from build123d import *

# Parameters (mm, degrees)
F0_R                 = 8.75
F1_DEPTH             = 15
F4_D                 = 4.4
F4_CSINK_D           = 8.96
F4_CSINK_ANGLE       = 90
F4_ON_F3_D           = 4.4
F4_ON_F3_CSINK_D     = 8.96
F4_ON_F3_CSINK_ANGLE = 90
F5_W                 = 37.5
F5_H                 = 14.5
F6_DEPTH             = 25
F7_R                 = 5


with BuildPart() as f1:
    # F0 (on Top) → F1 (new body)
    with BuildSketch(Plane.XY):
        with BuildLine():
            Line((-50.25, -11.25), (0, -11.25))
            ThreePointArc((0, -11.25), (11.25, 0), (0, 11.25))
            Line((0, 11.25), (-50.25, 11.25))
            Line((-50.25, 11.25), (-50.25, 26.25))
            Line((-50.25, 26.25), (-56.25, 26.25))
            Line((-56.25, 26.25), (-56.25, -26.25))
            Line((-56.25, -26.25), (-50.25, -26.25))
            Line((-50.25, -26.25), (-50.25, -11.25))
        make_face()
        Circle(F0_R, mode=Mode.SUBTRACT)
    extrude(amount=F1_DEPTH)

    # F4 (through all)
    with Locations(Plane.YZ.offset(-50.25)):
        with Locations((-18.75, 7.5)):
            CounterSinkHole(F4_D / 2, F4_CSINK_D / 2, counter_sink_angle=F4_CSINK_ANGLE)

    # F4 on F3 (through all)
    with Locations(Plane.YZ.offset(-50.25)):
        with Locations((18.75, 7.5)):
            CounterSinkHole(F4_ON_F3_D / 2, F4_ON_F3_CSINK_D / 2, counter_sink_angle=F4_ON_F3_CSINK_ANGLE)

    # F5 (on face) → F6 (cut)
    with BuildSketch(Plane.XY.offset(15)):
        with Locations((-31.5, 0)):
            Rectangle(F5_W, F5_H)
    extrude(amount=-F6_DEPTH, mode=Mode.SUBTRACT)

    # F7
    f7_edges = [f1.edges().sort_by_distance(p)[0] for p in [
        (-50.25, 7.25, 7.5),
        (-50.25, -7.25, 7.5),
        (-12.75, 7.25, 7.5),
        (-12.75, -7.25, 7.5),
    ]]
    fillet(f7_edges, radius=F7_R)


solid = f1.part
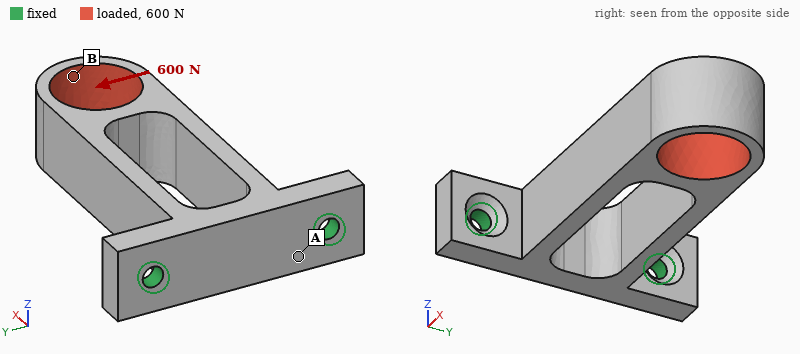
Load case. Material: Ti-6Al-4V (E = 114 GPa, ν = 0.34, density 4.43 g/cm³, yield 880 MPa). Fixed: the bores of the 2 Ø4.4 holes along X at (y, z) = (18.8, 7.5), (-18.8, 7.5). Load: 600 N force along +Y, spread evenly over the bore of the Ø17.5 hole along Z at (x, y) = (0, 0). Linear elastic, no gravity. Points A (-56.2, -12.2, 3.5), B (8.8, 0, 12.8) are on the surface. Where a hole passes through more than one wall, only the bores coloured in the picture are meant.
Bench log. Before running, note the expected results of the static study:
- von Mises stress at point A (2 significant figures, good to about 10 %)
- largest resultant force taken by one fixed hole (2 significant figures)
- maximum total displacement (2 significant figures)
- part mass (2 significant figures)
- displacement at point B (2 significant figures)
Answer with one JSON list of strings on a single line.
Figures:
["32 MPa", "1.1 kN", "0.20 mm", "57 g", "0.20 mm"]
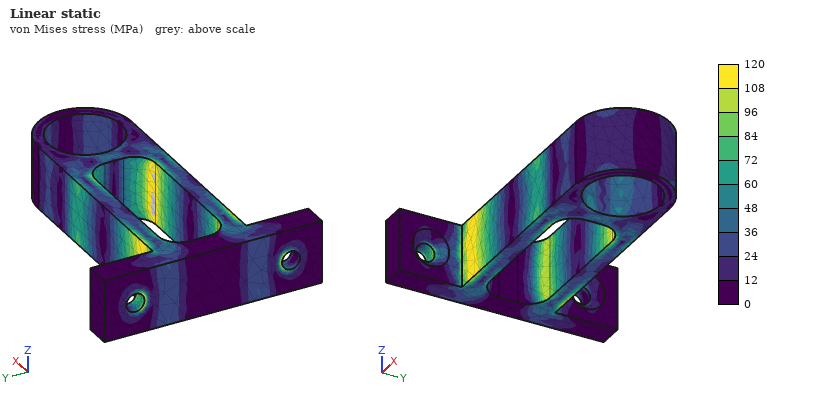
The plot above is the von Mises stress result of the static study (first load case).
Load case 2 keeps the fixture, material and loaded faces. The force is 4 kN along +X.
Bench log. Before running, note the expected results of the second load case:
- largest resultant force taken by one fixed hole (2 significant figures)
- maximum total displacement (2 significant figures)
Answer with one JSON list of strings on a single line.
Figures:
["2.3 kN", "47 µm"]
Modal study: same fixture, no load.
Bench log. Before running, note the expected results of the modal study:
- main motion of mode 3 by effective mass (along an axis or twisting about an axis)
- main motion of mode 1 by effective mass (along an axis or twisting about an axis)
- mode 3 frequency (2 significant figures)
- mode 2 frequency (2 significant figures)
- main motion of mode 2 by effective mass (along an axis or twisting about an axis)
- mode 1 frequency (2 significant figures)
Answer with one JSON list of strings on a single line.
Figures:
["twisting about X", "along Z", "4700 Hz", "2000 Hz", "along Y", "1500 Hz"]
